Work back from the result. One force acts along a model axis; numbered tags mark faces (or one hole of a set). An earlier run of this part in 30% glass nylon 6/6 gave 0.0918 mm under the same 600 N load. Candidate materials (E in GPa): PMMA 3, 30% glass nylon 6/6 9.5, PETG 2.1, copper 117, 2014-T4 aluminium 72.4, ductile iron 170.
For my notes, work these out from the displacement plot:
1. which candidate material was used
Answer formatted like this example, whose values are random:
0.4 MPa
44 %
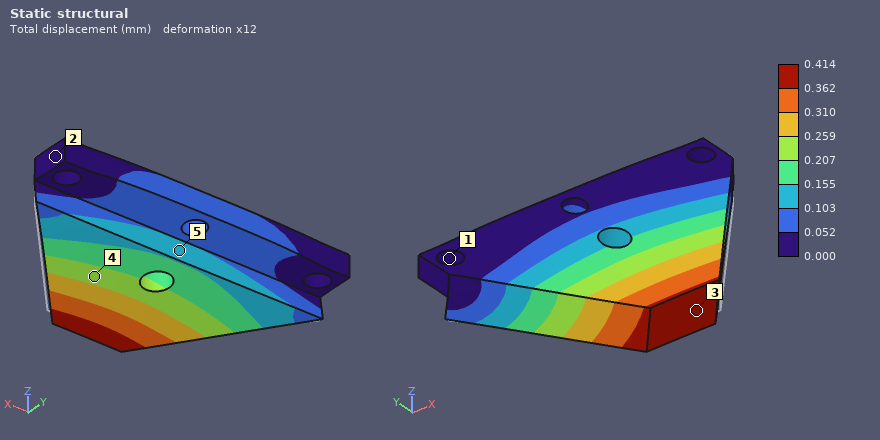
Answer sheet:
PETG
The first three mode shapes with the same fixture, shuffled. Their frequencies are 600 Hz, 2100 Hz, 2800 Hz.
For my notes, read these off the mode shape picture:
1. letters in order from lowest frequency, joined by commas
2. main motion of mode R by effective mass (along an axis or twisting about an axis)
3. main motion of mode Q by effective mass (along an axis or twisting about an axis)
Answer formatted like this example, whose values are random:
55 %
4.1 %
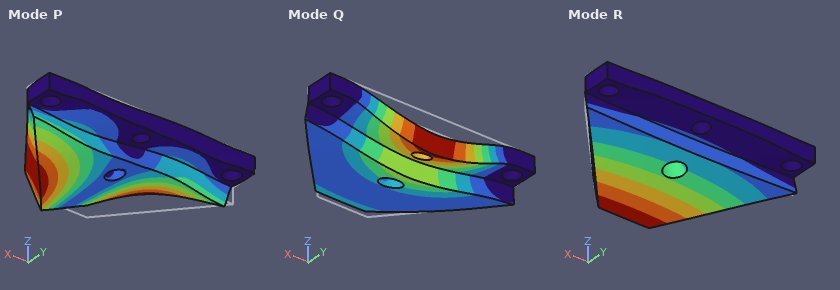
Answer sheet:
R, Q, P
along Z
along Z
